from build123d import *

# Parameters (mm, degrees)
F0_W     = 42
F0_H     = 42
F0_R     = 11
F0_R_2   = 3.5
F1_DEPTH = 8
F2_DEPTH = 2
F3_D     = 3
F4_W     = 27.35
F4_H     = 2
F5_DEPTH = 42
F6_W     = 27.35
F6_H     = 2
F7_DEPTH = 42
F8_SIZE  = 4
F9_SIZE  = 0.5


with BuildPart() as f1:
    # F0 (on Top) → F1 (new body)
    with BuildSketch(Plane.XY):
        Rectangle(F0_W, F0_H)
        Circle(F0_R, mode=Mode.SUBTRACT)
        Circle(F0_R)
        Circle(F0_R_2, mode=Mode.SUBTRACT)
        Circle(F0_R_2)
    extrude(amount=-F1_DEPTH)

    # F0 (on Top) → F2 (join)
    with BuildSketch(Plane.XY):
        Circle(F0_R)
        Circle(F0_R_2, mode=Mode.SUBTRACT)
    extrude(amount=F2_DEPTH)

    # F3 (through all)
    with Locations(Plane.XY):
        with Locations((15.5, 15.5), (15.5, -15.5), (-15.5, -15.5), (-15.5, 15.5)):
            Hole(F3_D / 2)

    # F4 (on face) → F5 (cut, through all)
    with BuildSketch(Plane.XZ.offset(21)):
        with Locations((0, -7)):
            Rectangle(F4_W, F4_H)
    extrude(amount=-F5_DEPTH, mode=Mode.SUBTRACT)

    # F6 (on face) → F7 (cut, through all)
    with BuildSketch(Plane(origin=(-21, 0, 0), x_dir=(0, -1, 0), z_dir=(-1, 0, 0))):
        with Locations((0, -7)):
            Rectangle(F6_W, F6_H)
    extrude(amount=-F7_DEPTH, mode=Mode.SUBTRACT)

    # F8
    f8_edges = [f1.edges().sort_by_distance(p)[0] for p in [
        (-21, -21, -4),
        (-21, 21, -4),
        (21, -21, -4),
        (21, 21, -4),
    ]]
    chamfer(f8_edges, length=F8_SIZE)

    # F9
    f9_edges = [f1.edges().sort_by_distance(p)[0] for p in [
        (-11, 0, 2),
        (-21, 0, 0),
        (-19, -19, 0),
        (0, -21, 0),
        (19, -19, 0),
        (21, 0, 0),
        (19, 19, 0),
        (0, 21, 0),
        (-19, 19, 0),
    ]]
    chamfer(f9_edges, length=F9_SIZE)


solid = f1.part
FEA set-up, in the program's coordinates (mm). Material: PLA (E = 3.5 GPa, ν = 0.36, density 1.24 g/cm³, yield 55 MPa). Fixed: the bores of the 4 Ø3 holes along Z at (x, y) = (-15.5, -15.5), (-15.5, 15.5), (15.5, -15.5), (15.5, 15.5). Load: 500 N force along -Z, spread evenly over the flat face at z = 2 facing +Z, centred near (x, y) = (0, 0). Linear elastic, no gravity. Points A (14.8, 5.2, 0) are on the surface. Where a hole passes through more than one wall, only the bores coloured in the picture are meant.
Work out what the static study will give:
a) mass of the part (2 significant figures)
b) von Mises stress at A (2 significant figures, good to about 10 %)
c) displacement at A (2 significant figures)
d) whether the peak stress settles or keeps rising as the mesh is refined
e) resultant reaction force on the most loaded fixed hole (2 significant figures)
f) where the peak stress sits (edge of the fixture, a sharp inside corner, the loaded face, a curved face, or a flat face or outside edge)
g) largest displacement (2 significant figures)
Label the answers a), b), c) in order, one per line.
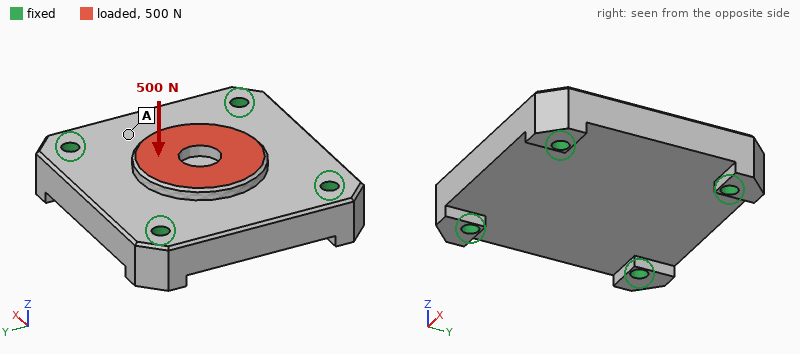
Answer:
a) 14 g
b) 2.3 MPa
c) 27 µm
d) keeps rising
e) 130 N
f) edge of the fixture
g) 61 µm
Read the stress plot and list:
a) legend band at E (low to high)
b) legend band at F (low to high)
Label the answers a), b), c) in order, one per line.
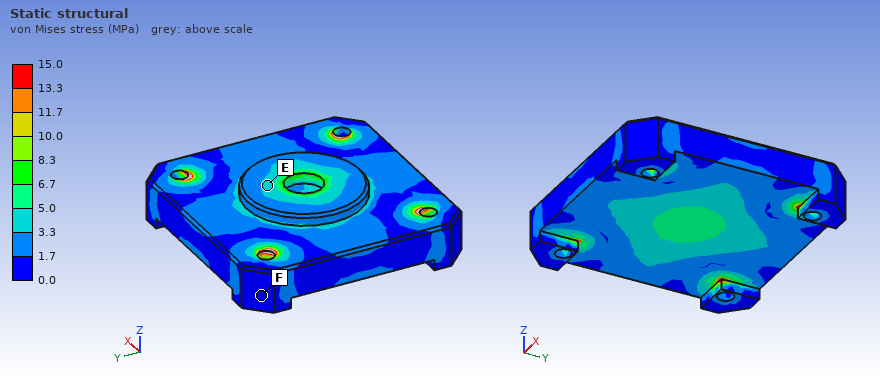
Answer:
a) 3.3 to 5.0 MPa
b) 0.0 to 1.7 MPa
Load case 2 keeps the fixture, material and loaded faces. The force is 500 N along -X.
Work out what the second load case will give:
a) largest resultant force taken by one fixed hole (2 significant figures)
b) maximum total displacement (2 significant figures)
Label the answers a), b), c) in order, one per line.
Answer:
a) 140 N
b) 23 µm
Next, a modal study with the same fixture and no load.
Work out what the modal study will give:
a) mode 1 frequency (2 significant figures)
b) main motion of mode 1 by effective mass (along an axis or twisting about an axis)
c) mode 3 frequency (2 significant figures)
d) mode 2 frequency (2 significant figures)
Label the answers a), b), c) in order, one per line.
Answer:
a) 6400 Hz
b) along Z
c) 9600 Hz
d) 9600 Hz
